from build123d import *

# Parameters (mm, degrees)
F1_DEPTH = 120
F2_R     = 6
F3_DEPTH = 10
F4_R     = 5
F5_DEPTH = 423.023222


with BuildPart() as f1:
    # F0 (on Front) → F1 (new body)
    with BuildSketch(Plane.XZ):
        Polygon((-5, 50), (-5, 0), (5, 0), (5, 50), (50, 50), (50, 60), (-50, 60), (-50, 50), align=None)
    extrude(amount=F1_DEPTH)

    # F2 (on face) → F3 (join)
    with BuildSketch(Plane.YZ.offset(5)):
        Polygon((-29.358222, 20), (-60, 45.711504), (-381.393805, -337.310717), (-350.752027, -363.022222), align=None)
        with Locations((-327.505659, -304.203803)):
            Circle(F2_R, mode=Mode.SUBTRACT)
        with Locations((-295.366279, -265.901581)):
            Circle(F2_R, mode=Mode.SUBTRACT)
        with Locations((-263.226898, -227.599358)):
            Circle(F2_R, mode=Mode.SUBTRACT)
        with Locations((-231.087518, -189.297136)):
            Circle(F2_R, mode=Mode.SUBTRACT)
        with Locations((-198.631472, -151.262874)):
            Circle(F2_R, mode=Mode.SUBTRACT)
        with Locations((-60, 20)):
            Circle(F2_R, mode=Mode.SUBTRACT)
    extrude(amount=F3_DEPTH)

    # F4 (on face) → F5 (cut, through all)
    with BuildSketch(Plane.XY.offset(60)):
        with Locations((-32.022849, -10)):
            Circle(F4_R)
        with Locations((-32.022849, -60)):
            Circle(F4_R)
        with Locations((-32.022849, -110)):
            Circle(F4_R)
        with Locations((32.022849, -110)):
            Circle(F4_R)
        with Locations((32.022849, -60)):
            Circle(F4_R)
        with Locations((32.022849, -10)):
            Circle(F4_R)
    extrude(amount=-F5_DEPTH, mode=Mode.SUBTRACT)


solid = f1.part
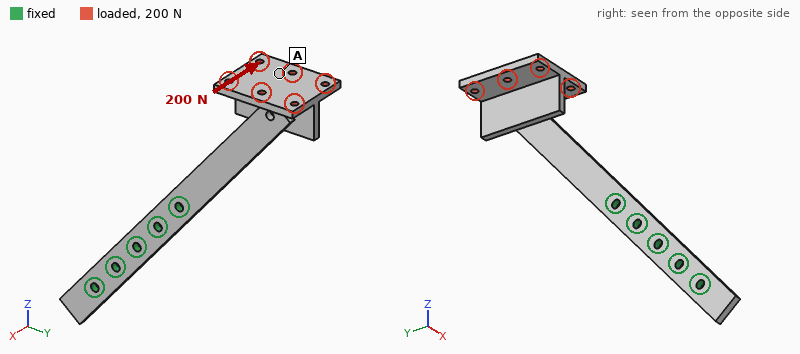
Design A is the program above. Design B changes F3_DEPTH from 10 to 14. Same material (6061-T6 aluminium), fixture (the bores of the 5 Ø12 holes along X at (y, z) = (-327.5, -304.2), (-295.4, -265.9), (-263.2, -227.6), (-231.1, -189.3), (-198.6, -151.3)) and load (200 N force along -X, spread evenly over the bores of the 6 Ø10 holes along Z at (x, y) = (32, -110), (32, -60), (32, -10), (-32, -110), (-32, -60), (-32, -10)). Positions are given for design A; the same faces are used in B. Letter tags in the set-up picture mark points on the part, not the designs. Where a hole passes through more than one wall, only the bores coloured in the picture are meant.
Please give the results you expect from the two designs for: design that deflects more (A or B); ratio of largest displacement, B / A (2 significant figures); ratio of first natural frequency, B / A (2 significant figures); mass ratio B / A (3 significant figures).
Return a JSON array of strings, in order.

["A", "0.37", "1.6", "1.21"]
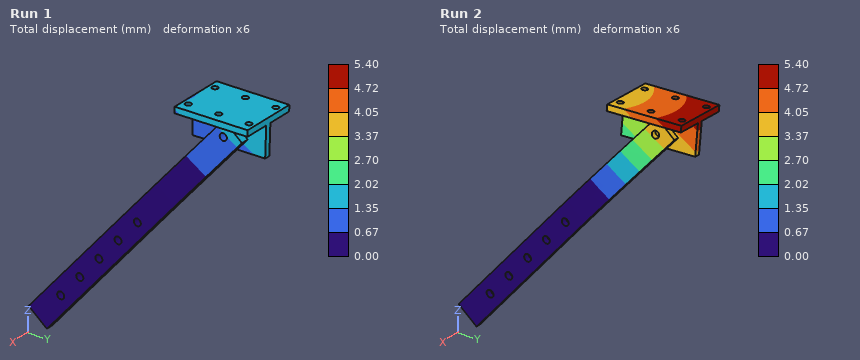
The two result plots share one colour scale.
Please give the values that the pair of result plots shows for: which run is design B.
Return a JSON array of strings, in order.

["Run 1"]
